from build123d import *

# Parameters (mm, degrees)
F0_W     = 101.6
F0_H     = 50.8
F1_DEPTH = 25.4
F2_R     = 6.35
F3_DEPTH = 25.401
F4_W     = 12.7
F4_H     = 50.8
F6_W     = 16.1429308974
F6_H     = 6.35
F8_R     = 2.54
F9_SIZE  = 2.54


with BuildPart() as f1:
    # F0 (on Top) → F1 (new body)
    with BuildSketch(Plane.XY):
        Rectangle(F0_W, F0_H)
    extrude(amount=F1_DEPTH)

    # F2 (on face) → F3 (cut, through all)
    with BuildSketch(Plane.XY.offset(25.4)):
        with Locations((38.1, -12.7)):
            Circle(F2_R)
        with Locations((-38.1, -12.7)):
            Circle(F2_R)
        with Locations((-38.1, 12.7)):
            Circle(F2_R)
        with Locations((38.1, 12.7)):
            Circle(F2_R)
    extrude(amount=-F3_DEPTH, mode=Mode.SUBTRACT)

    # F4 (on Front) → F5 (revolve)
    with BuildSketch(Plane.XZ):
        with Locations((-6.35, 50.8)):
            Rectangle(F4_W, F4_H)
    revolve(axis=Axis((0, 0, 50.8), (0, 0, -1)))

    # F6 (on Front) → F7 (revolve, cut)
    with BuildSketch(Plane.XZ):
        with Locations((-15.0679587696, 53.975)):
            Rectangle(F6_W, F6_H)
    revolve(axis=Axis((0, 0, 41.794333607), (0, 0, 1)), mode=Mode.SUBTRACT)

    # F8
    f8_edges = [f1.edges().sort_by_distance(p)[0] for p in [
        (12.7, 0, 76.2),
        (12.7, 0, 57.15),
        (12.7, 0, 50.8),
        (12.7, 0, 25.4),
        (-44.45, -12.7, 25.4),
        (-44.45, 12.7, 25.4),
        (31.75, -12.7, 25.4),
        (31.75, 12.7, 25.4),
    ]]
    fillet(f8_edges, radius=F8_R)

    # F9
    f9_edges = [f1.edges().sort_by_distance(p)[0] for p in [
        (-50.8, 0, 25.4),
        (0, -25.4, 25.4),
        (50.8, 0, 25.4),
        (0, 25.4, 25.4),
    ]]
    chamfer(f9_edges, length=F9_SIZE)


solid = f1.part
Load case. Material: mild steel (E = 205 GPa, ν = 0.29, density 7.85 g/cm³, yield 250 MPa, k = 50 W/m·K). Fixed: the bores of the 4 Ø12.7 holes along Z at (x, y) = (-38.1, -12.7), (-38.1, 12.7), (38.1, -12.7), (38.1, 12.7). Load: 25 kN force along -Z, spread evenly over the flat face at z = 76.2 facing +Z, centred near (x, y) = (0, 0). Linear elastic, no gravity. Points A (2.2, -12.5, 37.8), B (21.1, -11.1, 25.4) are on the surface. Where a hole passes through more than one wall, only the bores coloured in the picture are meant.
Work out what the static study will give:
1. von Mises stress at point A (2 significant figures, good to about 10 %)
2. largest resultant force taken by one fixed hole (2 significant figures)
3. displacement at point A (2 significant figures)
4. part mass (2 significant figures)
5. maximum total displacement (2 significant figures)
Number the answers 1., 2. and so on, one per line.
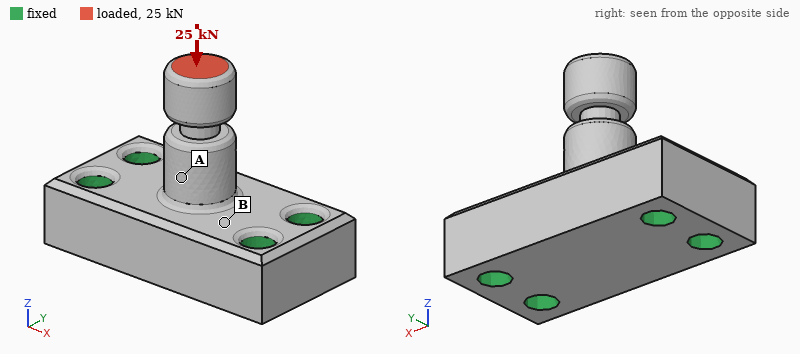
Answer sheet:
1. 43 MPa
2. 6.4 kN
3. 9.9 µm
4. 1.1 kg
5. 28 µm
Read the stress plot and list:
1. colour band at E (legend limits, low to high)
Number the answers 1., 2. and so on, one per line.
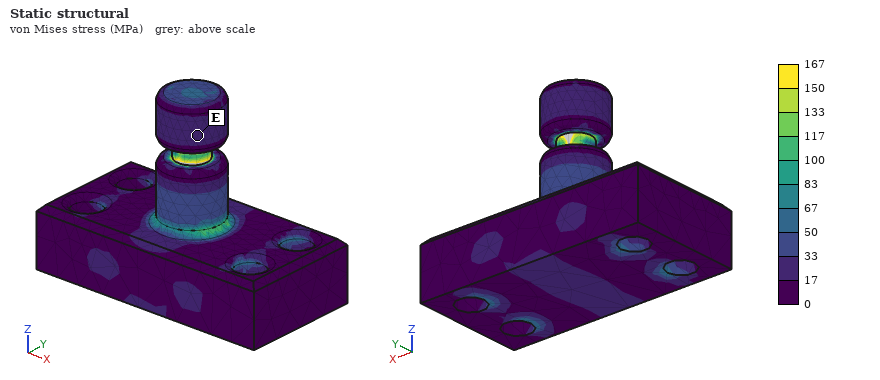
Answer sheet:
1. 17 to 33 MPa
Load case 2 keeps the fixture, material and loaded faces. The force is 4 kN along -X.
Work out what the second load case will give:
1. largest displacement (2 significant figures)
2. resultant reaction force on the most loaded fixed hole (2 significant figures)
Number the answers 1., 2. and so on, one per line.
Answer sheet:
1. 0.12 mm
2. 2.5 kN
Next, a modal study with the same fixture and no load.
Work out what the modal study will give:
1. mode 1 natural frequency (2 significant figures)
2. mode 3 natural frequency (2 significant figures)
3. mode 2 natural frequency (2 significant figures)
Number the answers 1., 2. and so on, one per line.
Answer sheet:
1. 4300 Hz
2. 10000 Hz
3. 4500 Hz
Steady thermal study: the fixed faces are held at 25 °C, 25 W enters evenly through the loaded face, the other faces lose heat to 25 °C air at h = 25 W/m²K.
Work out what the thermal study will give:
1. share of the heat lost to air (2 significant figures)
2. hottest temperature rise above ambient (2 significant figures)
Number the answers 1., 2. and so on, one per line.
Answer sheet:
1. 20 %
2. 77 K
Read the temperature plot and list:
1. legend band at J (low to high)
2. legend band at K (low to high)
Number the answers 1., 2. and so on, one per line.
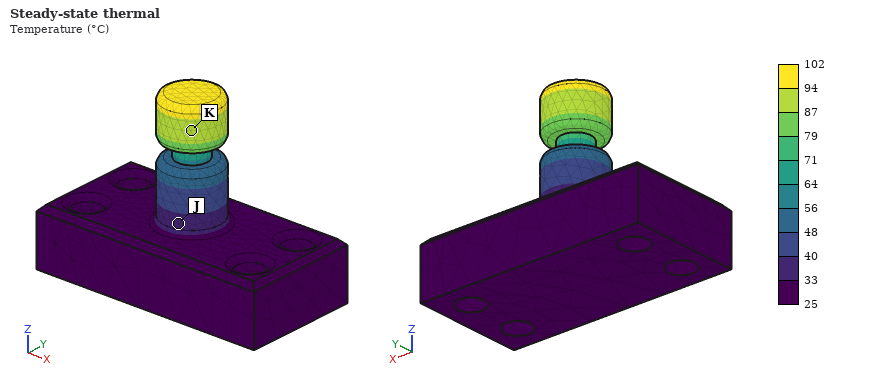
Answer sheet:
1. 33 to 40 °C
2. 87 to 94 °C
